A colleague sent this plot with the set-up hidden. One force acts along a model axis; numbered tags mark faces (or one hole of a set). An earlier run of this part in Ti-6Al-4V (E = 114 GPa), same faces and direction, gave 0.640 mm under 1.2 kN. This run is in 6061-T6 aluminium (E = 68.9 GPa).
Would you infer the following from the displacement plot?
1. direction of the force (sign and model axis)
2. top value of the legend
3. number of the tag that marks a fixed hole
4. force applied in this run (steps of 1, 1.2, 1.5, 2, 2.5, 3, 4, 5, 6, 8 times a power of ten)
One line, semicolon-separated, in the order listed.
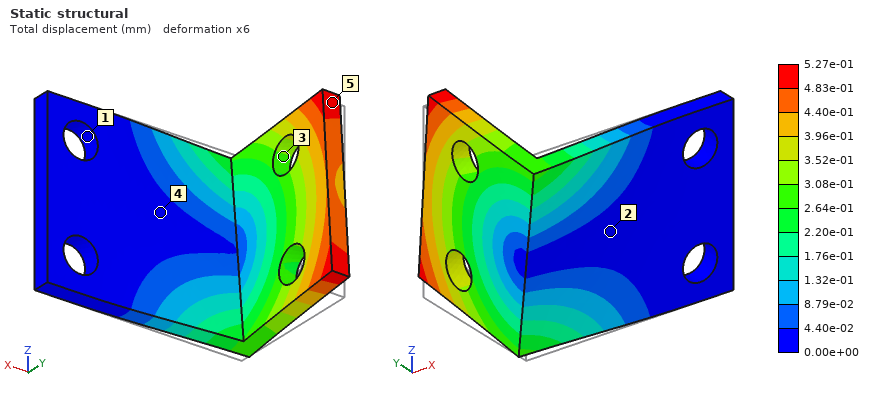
+Z; 5.27e-01 mm; 1; 600 N
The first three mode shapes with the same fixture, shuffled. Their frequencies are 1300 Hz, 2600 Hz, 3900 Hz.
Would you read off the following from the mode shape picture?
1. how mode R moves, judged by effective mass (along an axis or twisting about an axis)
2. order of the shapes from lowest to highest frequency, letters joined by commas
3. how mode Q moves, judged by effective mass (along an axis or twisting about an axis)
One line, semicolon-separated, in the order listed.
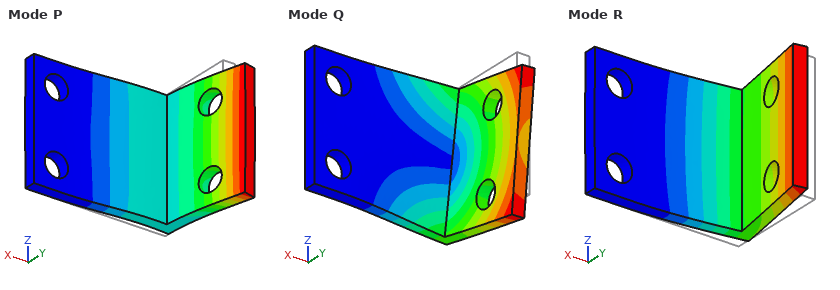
along Y; R, Q, P; along Z
